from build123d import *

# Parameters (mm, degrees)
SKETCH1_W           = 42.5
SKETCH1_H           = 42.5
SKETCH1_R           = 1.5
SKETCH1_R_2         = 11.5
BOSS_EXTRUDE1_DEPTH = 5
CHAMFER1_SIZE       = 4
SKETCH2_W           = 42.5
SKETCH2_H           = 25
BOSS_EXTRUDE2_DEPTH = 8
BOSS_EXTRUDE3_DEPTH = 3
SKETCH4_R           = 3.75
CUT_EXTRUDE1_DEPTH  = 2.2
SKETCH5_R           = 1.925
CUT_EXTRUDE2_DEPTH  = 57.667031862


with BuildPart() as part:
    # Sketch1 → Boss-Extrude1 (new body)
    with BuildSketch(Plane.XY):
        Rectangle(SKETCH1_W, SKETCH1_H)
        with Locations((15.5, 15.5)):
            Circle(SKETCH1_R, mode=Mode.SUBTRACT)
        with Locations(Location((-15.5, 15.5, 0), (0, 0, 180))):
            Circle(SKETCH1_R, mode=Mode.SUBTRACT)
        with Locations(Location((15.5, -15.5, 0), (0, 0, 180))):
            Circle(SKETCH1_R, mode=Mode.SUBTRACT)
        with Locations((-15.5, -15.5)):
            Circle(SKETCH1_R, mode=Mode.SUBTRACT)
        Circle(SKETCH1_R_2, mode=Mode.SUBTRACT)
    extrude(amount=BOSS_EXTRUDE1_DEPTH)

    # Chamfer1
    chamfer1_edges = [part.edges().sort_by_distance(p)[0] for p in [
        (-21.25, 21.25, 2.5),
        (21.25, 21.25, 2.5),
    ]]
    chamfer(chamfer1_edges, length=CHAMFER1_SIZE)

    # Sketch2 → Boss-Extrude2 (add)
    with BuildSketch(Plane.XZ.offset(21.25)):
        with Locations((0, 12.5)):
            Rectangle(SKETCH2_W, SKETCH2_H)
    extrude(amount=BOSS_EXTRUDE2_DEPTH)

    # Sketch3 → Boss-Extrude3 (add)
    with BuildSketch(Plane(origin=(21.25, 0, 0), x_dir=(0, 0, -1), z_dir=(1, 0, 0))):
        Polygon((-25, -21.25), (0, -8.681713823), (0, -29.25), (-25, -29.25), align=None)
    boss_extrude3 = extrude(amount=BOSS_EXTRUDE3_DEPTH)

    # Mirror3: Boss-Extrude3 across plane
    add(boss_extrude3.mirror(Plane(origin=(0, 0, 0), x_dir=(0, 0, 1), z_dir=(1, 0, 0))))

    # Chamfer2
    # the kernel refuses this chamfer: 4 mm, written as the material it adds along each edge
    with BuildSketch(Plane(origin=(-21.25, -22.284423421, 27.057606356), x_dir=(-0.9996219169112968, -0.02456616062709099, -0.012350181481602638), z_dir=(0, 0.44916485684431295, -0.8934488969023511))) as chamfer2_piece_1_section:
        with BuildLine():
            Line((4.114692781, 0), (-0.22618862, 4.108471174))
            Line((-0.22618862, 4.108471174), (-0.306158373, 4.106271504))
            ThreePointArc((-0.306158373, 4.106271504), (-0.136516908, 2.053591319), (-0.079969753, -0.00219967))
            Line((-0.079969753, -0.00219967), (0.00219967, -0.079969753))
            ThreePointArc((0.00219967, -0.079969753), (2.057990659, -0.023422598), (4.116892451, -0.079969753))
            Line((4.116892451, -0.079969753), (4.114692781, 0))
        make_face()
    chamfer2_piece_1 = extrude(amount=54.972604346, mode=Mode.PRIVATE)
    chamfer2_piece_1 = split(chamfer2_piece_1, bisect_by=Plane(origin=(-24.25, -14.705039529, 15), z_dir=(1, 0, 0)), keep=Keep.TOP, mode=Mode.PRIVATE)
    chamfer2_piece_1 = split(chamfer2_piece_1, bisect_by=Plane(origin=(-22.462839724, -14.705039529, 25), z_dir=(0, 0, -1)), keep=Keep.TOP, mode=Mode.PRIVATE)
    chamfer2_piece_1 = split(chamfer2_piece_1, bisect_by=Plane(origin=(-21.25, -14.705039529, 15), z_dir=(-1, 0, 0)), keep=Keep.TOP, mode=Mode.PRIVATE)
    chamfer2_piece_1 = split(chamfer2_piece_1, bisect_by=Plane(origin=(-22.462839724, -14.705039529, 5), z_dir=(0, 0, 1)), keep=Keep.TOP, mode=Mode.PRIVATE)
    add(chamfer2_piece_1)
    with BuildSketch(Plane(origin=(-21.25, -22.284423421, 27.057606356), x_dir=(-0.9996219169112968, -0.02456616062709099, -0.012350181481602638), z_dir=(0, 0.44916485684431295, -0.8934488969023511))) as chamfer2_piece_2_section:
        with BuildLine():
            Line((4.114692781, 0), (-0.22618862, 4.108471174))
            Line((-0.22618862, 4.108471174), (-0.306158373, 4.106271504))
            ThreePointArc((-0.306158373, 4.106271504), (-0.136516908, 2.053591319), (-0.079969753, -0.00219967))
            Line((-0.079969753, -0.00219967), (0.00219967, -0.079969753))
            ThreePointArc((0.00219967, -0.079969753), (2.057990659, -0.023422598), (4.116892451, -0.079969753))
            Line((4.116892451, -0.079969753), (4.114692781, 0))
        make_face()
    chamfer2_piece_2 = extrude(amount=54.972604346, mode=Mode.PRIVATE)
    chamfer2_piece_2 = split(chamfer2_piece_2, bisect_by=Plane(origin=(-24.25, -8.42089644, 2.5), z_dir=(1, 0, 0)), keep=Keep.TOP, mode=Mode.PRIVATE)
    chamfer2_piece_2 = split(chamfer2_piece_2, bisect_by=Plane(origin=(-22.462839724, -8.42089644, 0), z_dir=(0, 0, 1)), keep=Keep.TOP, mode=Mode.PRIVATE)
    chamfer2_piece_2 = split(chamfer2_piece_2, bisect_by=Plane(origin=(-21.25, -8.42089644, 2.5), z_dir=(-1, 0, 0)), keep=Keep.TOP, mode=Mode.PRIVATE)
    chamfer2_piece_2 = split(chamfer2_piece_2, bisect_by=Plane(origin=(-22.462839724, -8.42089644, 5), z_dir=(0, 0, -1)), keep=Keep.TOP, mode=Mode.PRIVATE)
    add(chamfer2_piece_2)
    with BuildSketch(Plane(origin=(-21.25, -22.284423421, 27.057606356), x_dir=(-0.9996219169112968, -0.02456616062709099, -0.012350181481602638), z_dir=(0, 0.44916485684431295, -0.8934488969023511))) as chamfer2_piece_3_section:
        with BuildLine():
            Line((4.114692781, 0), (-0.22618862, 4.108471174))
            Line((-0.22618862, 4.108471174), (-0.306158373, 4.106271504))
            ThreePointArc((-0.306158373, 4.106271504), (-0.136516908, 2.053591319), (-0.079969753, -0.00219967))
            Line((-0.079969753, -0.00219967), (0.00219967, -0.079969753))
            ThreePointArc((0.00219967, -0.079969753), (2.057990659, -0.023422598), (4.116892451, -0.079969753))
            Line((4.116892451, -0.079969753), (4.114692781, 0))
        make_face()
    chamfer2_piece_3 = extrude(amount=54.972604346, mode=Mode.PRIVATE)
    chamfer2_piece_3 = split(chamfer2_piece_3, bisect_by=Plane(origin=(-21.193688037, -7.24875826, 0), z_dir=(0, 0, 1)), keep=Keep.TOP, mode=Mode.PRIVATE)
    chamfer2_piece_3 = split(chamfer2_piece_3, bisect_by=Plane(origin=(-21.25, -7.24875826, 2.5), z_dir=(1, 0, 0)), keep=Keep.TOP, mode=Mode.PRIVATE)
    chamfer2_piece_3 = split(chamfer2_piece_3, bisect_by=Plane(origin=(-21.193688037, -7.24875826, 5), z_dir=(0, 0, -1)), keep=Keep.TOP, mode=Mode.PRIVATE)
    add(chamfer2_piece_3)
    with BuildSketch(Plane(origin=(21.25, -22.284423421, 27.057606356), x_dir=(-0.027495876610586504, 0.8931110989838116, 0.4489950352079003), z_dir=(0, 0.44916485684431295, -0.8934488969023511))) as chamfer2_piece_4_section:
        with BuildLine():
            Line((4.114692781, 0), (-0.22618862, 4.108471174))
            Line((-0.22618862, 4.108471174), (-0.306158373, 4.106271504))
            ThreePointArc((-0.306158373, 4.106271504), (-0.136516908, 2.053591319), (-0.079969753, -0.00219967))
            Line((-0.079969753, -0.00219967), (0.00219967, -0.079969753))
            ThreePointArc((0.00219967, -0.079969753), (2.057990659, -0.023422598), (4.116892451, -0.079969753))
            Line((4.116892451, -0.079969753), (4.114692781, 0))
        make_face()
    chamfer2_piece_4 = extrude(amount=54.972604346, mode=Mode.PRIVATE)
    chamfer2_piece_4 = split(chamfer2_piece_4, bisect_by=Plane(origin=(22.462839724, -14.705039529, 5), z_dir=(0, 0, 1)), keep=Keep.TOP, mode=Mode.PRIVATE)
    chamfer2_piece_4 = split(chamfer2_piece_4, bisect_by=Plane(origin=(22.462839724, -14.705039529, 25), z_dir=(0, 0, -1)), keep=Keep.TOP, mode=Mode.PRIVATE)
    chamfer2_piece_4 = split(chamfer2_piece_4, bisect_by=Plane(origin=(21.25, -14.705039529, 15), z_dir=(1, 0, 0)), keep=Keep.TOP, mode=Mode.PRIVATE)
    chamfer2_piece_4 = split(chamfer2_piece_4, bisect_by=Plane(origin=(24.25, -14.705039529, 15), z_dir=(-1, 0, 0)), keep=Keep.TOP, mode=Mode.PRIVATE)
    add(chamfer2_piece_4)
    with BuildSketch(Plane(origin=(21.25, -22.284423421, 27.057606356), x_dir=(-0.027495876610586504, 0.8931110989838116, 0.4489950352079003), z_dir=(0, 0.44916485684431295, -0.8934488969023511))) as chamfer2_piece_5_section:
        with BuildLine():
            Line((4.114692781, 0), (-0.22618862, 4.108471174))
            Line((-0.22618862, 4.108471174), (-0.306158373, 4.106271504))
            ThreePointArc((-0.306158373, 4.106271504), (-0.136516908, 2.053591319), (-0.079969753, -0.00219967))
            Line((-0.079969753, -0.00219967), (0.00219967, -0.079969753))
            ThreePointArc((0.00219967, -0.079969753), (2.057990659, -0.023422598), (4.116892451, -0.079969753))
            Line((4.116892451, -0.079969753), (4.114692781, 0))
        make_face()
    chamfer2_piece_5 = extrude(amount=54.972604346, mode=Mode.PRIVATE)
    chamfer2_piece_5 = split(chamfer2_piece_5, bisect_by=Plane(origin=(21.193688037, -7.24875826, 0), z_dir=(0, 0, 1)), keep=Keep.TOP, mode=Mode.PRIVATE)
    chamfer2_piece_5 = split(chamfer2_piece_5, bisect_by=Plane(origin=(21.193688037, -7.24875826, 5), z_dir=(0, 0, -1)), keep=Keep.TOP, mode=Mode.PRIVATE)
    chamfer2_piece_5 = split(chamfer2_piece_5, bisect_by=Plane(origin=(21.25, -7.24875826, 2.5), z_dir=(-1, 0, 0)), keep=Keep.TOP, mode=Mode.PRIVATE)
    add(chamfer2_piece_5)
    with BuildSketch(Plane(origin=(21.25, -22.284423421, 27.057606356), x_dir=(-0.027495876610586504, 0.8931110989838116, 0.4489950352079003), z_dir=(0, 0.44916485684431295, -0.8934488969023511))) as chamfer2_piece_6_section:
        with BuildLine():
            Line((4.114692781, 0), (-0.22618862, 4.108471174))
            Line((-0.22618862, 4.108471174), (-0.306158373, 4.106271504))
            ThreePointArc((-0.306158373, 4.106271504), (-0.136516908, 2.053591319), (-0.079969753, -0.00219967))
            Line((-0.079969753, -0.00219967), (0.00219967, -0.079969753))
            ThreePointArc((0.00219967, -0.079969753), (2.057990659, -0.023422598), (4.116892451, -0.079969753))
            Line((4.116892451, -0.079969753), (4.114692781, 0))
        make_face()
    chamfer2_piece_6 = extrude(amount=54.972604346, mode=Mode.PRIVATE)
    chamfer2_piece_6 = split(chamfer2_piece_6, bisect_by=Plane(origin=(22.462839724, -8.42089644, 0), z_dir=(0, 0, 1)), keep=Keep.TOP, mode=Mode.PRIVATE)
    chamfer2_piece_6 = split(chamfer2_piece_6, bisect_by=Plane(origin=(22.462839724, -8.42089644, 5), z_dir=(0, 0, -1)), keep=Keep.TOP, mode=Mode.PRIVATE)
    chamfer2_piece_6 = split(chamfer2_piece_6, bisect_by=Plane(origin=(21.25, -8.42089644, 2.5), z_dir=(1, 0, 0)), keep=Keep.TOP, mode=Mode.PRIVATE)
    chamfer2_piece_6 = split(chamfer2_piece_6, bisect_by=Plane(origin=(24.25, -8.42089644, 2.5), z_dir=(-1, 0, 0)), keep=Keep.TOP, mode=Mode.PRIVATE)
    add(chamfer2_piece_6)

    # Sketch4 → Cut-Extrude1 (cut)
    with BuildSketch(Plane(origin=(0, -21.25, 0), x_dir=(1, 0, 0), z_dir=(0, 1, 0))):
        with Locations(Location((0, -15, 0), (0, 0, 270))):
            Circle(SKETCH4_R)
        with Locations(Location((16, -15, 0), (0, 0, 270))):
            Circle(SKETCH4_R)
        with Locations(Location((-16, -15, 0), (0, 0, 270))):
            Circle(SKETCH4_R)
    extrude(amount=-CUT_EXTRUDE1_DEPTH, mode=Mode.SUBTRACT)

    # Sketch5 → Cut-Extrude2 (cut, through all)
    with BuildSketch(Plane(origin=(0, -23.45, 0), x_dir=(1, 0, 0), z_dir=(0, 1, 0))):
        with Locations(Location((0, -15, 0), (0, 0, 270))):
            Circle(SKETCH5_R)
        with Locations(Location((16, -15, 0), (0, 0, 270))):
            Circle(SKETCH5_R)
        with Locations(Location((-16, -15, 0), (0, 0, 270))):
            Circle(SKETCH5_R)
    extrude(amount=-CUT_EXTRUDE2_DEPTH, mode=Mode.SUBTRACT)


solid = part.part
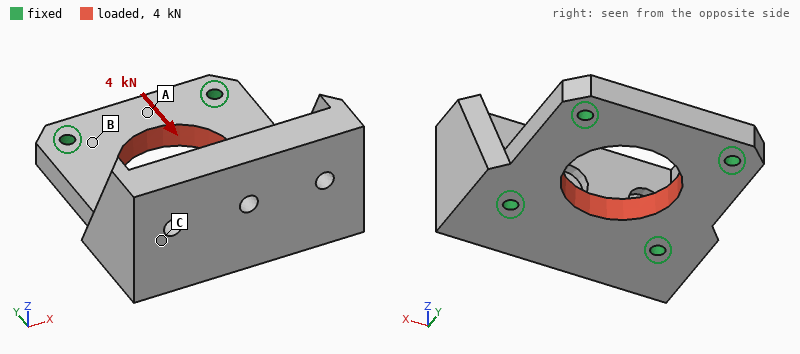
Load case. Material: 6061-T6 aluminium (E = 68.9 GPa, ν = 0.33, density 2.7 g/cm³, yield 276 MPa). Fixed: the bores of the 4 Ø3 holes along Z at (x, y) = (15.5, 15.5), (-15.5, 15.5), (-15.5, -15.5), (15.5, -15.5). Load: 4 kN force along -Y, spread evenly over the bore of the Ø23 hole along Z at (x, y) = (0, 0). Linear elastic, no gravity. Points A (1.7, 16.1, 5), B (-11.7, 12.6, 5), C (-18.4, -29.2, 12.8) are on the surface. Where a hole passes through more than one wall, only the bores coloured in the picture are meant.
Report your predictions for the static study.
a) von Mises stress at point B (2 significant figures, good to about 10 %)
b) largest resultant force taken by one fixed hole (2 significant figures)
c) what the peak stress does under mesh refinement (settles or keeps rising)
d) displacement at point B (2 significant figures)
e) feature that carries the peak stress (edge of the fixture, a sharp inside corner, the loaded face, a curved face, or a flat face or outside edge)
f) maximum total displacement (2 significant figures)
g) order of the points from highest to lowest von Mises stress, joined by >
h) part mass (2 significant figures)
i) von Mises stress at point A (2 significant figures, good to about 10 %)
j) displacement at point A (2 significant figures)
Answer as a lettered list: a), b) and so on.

a) 18 MPa
b) 1.0 kN
c) keeps rising
d) 2.5 µm
e) edge of the fixture
f) 8.2 µm
g) B > A > C
h) 47 g
i) 9.3 MPa
j) 7.6 µm
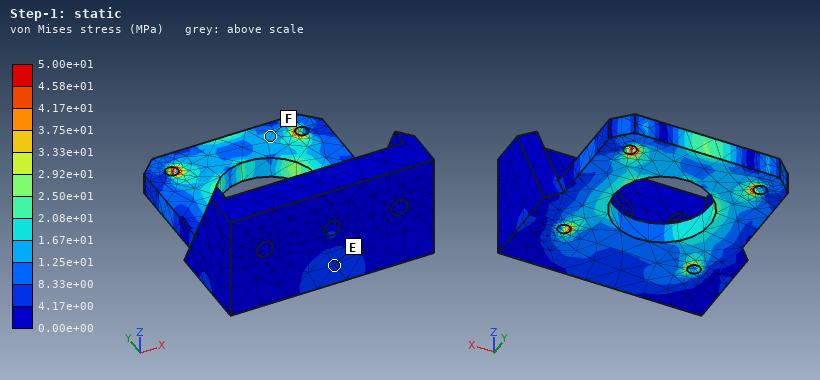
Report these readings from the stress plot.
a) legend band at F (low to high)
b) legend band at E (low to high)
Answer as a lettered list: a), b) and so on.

a) 1.25e+01 to 1.67e+01 MPa
b) 4.17e+00 to 8.33e+00 MPa
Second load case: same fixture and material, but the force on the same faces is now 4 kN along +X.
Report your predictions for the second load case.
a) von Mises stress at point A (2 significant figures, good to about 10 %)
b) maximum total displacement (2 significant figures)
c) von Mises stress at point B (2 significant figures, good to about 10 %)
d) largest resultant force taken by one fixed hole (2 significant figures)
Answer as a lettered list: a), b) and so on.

a) 14 MPa
b) 7.2 µm
c) 19 MPa
d) 1.1 kN
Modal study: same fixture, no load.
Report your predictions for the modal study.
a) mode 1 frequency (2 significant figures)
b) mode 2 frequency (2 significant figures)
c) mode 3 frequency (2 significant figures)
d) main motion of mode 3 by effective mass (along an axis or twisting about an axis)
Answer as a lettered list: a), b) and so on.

a) 5000 Hz
b) 8600 Hz
c) 15 kHz
d) along X
